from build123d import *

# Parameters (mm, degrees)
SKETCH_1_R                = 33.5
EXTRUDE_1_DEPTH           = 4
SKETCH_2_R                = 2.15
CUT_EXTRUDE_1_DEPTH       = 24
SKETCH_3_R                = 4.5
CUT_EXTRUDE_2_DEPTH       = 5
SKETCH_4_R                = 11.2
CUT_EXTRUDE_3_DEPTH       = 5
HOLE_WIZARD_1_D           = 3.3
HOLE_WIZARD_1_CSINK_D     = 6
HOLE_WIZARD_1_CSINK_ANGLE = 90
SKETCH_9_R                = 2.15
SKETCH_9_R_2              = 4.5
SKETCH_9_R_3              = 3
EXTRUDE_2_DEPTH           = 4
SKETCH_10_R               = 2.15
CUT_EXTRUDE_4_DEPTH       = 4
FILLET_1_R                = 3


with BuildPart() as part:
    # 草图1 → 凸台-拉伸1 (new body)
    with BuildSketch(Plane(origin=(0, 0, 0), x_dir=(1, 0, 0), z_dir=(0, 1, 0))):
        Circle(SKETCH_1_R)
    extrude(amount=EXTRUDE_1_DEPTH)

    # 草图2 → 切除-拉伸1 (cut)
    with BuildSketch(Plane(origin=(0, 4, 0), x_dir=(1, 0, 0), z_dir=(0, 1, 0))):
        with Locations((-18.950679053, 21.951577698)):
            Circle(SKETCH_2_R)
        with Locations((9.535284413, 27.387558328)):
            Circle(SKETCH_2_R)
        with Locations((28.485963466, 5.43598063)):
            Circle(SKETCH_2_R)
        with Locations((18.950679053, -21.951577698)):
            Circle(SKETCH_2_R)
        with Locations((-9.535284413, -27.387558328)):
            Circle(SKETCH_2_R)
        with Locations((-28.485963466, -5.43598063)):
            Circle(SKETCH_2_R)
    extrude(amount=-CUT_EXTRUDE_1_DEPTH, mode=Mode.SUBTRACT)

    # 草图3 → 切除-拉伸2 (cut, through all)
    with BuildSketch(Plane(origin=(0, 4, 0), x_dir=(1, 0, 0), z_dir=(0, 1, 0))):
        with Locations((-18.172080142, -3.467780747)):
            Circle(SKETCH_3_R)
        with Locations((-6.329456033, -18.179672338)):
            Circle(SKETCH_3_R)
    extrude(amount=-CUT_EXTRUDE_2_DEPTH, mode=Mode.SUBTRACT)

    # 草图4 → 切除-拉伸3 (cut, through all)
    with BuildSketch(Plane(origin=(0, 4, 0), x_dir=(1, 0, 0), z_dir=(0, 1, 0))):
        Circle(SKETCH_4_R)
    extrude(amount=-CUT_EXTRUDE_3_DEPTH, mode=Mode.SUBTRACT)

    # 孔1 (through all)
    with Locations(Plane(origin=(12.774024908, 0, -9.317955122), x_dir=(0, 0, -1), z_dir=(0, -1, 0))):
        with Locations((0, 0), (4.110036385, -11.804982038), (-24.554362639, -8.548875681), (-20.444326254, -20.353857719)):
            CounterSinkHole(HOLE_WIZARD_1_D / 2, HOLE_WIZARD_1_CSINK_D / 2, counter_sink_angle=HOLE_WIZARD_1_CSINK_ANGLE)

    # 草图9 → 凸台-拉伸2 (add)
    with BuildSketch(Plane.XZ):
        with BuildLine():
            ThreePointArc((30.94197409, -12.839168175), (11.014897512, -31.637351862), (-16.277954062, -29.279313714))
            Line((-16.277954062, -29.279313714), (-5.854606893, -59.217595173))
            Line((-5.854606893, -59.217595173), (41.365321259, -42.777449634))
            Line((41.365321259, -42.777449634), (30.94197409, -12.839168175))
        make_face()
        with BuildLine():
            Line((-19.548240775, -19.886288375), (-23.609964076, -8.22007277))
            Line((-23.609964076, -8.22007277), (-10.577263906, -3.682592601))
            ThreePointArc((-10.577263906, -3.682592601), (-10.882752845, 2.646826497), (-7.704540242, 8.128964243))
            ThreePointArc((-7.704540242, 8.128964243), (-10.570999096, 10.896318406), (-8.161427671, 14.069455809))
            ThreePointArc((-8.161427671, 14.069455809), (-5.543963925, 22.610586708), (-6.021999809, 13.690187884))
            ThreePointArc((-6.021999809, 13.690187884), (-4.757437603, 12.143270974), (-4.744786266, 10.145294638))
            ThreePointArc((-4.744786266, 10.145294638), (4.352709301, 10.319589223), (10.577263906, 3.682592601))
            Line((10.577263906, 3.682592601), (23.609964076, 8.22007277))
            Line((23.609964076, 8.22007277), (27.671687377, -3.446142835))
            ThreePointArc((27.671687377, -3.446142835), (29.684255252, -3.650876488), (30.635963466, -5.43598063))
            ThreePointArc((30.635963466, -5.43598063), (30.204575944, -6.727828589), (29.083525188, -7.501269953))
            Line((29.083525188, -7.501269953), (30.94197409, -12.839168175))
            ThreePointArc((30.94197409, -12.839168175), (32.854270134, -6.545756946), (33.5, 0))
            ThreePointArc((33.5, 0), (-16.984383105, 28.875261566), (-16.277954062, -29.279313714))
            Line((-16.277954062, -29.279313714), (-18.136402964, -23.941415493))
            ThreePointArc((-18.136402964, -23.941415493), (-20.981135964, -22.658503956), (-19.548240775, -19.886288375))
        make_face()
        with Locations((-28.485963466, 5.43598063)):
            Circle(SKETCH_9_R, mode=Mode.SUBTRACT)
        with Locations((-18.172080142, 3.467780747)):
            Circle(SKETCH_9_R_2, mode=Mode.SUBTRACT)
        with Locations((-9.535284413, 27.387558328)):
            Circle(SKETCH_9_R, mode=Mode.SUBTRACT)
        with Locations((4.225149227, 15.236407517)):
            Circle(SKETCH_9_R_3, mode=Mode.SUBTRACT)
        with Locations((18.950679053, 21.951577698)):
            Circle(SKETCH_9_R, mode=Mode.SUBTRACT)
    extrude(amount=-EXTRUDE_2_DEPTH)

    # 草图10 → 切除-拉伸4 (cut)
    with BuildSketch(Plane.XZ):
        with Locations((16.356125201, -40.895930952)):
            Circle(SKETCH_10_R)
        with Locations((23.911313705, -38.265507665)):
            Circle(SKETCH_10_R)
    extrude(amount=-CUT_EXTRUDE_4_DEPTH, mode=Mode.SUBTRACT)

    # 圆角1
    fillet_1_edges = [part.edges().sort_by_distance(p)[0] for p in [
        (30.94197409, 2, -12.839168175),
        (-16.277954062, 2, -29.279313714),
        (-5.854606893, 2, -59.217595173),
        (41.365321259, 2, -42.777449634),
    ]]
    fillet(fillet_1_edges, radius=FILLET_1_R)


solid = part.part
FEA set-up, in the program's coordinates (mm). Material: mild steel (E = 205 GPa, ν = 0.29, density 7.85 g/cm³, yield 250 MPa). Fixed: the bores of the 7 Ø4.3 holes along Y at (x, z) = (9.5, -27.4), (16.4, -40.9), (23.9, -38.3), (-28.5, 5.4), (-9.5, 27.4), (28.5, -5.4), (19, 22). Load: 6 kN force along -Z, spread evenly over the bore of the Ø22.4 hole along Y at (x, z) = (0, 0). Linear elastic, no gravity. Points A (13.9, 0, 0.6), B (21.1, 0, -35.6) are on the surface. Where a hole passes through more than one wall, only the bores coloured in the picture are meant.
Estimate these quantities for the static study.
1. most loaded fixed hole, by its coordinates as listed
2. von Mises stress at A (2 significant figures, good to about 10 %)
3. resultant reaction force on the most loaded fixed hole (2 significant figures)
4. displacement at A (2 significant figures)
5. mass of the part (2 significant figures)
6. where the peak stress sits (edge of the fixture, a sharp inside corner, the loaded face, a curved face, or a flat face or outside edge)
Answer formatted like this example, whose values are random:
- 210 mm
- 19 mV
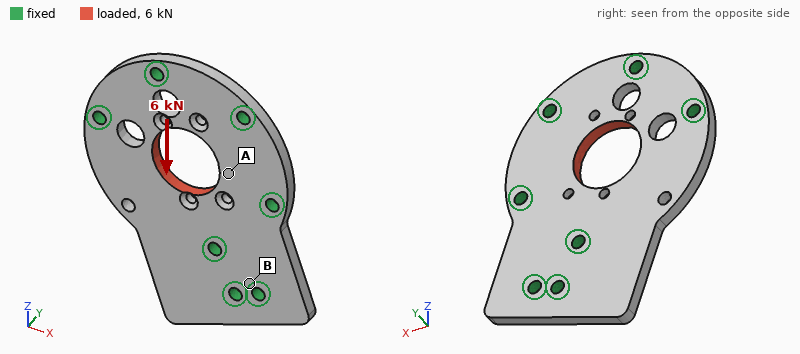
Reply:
- (9.5, -27.4)
- 28 MPa
- 1.6 kN
- 1.9 µm
- 130 g
- the loaded face
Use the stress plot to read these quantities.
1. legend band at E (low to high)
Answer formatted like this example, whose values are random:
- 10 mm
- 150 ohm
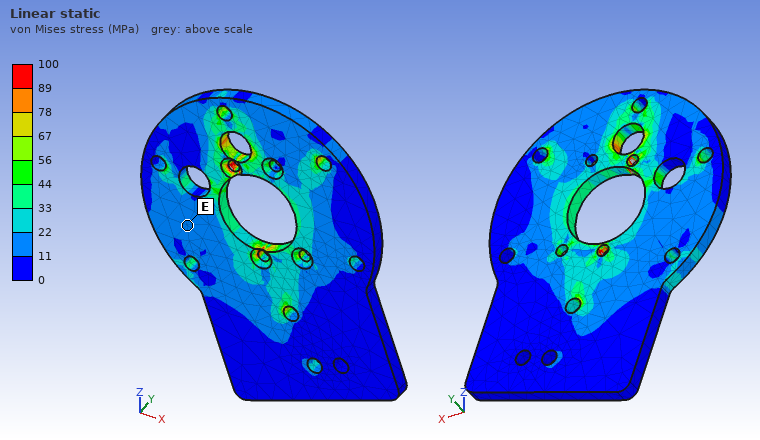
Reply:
- 11 to 22 MPa
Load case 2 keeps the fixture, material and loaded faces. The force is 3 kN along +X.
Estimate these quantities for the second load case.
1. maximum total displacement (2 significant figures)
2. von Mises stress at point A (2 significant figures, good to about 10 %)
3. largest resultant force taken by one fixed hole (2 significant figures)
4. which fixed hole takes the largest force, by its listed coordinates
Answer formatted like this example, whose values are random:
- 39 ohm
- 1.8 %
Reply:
- 3.1 µm
- 11 MPa
- 860 N
- (28.5, -5.4)
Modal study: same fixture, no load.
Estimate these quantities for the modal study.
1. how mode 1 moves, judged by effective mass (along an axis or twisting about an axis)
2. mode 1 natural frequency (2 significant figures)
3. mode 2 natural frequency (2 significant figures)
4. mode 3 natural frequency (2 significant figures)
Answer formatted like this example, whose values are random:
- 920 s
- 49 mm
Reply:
- along Y
- 5200 Hz
- 7500 Hz
- 12 kHz
